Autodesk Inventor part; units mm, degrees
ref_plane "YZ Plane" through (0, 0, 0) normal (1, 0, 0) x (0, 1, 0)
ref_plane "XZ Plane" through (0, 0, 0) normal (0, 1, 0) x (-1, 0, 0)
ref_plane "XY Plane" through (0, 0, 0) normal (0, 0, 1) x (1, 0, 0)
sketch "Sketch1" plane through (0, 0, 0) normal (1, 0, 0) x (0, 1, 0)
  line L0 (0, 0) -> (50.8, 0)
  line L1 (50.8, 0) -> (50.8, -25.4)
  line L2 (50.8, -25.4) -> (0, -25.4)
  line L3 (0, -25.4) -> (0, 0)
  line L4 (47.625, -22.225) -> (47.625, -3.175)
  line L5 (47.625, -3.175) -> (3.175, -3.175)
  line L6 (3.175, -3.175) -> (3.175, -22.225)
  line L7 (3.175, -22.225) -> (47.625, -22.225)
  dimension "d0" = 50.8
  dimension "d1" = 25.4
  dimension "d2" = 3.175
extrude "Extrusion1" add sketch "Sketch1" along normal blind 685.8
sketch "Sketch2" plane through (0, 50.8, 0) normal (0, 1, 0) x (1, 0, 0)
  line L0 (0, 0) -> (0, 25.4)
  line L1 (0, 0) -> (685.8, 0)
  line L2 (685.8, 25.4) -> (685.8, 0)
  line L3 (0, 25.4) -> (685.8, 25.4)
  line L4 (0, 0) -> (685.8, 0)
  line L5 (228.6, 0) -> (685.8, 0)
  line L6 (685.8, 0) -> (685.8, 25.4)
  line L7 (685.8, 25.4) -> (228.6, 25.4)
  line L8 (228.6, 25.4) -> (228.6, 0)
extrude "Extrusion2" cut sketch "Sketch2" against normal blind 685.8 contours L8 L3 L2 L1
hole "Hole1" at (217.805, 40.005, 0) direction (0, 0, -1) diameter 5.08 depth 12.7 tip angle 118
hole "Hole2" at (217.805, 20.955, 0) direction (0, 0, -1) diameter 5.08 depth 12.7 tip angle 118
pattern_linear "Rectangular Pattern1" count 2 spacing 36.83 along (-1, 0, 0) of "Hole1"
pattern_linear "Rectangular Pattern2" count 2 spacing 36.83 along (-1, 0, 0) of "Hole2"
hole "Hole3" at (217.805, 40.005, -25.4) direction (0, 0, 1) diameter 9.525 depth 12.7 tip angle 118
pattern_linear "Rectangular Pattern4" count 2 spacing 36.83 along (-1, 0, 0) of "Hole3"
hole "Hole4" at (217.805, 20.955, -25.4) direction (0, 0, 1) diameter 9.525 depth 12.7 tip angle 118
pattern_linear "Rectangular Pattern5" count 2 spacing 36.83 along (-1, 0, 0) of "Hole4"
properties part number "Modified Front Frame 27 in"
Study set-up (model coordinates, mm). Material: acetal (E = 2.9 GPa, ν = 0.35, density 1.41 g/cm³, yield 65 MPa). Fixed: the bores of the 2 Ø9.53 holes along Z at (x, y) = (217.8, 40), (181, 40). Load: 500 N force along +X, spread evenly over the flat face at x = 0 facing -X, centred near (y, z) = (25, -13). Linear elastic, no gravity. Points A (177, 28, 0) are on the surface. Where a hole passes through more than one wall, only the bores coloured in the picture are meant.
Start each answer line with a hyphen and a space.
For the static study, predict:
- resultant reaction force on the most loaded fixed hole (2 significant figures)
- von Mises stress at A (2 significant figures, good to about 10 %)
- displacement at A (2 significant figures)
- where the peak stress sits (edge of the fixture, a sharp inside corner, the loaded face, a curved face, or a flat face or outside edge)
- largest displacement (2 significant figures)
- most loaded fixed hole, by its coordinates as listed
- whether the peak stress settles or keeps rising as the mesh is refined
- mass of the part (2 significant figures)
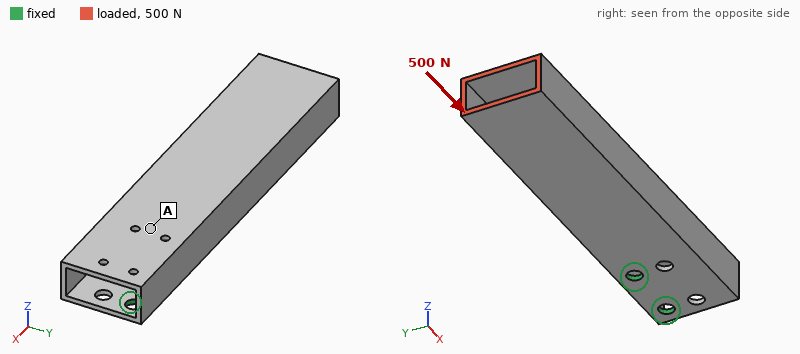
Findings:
- 350 N
- 1.6 MPa
- 0.20 mm
- edge of the fixture
- 1.3 mm
- (181, 40)
- keeps rising
- 140 g
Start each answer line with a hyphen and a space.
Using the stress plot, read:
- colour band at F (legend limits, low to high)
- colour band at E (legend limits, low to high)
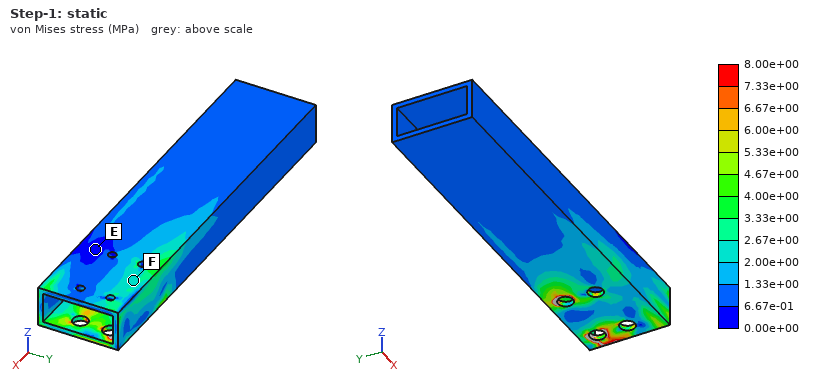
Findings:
- 2.00e+00 to 2.67e+00 MPa
- 0.00e+00 to 6.67e-01 MPa
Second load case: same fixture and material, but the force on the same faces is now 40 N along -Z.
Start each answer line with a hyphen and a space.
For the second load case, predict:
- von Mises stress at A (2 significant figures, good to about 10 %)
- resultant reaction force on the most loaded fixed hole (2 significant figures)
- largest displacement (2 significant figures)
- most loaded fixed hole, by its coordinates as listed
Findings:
- 2.2 MPa
- 240 N
- 2.5 mm
- (181, 40)
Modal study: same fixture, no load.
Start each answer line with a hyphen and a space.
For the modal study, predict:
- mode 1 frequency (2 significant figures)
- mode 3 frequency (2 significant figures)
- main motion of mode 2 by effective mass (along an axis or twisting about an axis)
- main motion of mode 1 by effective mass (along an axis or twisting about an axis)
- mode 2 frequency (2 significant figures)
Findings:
- 100 Hz
- 260 Hz
- along Y
- along Z
- 180 Hz
